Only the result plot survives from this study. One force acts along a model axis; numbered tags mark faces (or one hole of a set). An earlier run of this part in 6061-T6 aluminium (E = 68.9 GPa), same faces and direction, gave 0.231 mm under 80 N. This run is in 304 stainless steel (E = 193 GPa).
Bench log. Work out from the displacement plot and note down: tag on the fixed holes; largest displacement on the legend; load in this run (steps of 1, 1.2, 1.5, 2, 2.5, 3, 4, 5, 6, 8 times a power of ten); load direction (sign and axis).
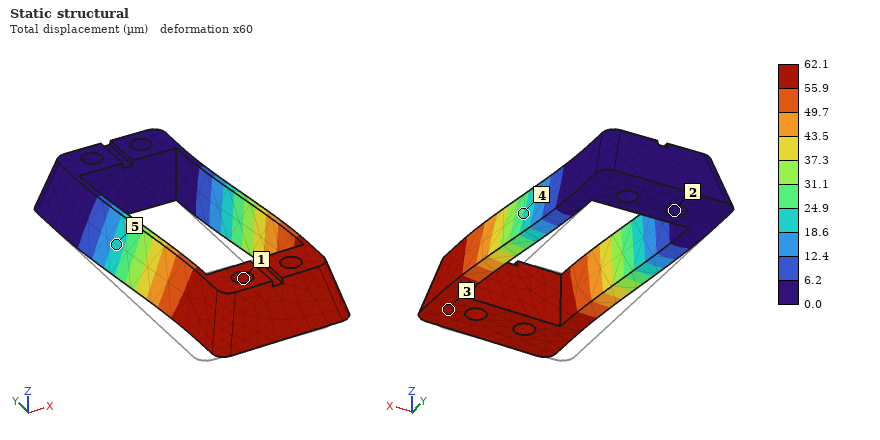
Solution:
2
62.1 µm
60 N
+X
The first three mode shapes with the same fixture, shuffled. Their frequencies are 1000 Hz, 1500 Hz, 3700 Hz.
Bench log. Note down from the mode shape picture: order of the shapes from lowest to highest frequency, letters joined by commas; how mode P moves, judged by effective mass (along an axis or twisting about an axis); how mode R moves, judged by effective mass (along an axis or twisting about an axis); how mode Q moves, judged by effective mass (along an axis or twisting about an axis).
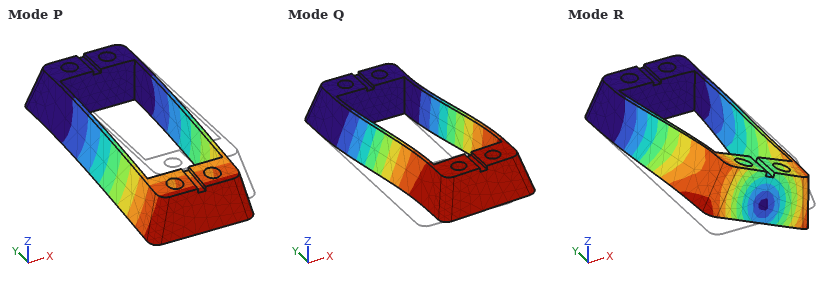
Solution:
Q, P, R
along Z
twisting about Y
along X
